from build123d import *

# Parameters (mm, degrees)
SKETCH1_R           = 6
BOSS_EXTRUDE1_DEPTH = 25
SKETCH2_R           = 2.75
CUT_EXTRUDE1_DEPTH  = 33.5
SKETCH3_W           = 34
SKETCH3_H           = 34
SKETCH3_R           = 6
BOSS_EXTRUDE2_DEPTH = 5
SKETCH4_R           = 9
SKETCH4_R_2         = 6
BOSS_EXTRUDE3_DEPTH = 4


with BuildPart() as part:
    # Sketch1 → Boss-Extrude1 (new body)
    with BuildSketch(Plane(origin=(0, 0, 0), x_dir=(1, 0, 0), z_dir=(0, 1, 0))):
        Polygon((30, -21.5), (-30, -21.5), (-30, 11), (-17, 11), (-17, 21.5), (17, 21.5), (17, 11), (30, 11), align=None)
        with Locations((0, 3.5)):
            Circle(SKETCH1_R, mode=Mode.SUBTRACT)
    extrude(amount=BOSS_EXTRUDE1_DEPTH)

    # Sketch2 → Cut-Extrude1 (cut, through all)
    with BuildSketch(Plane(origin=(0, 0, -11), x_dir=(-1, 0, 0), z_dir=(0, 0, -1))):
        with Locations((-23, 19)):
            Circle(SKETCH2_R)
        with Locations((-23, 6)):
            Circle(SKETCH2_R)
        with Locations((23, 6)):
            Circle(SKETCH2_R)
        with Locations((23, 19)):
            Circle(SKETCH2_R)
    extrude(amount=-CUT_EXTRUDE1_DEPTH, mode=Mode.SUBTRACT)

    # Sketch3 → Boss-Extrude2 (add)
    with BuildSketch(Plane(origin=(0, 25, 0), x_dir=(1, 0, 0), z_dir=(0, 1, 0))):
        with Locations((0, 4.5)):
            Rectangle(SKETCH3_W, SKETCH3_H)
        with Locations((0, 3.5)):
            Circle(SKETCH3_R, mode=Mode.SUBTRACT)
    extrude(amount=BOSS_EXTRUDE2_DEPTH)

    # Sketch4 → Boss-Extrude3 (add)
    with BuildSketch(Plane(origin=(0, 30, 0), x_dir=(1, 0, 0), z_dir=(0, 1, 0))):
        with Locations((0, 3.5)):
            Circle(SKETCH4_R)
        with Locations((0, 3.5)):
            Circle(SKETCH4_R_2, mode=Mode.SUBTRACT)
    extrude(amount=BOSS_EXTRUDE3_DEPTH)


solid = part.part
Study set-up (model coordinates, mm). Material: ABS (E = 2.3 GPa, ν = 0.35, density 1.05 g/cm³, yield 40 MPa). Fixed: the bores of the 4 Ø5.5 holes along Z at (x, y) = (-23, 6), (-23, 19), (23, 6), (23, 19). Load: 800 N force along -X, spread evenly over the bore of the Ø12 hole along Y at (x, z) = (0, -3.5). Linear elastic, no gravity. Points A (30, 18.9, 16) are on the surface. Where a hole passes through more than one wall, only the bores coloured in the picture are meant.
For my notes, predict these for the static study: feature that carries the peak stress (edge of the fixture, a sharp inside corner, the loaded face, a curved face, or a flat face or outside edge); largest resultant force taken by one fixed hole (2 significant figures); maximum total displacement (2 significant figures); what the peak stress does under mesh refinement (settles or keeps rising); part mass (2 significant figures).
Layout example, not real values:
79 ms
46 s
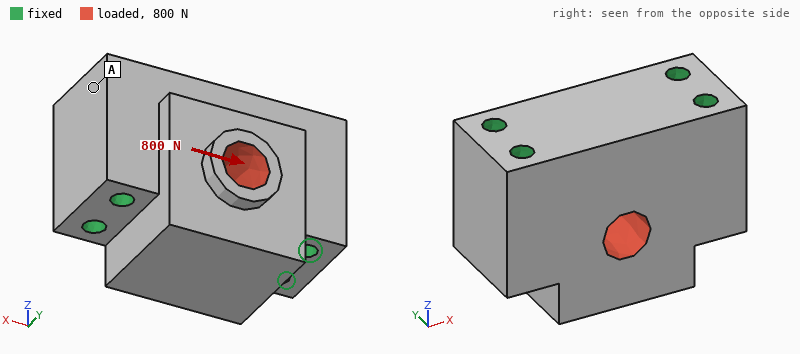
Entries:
edge of the fixture
240 N
15 µm
keeps rising
60 g
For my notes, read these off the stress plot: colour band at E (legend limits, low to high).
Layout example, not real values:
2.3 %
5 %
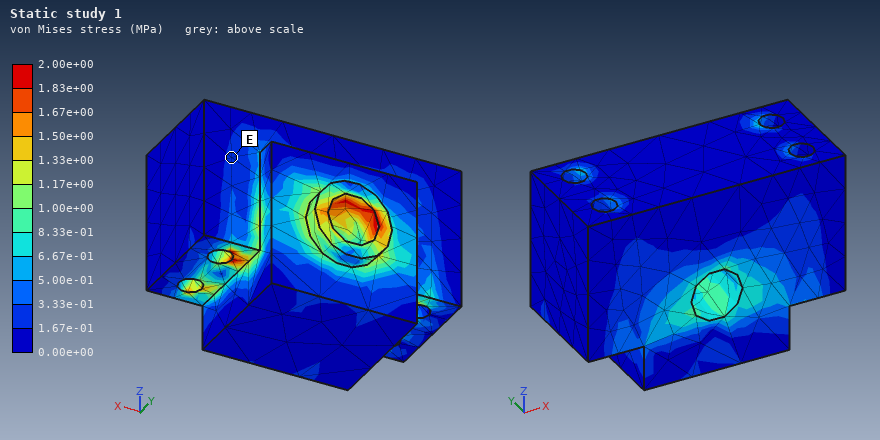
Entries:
1.67e-01 to 3.33e-01 MPa
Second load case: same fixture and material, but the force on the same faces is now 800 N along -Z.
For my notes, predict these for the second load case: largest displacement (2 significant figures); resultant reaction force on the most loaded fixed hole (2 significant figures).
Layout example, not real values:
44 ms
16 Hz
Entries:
25 µm
260 N
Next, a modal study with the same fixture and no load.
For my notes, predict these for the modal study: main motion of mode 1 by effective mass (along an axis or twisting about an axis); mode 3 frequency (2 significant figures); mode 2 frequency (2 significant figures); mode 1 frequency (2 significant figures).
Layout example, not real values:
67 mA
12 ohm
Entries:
along Y
8800 Hz
8300 Hz
5600 Hz
